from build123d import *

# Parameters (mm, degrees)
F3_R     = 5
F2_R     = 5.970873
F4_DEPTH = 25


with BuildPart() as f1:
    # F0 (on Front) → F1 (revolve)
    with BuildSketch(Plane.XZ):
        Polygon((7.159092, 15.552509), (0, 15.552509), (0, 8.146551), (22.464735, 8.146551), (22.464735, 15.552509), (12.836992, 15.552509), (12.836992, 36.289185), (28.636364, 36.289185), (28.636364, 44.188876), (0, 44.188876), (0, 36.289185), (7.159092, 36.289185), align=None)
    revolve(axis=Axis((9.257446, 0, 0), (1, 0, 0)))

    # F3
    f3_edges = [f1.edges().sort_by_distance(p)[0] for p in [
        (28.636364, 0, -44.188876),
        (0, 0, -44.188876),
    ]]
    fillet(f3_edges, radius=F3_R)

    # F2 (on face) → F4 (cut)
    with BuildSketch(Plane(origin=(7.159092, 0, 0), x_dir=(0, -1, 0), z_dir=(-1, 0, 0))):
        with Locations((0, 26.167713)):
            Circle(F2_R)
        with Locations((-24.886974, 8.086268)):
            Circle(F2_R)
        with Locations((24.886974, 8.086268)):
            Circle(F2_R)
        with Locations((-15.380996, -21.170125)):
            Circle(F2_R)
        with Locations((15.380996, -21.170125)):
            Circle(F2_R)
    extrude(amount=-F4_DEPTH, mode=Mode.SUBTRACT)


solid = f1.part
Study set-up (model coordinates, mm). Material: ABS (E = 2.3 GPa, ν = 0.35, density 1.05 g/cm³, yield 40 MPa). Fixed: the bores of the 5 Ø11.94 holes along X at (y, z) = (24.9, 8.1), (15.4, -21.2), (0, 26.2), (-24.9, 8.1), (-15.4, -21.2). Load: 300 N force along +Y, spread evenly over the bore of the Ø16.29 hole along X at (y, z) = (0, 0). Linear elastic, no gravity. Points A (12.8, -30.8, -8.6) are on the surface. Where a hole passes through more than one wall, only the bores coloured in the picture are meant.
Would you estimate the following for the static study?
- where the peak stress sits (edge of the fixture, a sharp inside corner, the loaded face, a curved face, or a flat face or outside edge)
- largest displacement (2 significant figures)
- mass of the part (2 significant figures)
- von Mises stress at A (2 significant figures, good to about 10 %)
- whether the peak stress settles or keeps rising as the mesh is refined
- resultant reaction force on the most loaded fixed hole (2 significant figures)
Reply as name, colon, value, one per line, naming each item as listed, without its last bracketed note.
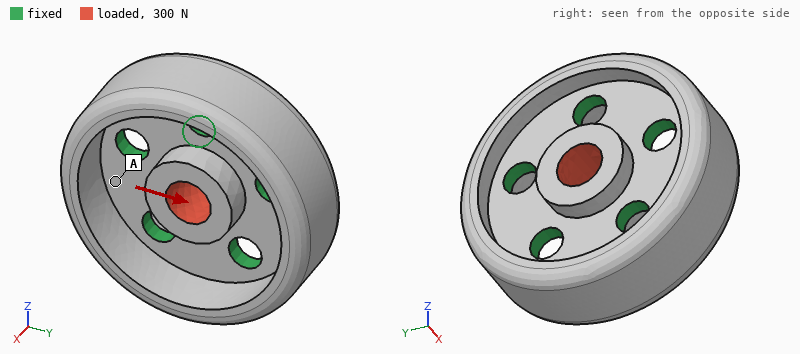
where the peak stress sits: edge of the fixture
largest displacement: 7.6 µm
mass of the part: 87 g
von Mises stress at A: 0.13 MPa
whether the peak stress settles or keeps rising as the mesh is refined: keeps rising
resultant reaction force on the most loaded fixed hole: 85 N
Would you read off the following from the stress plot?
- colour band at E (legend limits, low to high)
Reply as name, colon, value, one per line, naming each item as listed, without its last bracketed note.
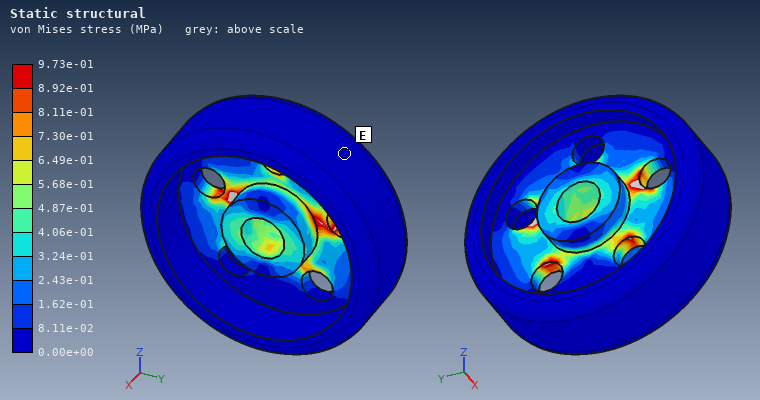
colour band at E: 0.00e+00 to 8.11e-02 MPa
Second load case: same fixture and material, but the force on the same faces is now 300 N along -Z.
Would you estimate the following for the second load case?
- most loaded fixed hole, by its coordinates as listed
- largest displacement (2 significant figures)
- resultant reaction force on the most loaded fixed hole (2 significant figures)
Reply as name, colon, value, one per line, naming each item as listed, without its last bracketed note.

most loaded fixed hole, by its coordinates as listed: (0, 26.2)
largest displacement: 7.6 µm
resultant reaction force on the most loaded fixed hole: 89 N
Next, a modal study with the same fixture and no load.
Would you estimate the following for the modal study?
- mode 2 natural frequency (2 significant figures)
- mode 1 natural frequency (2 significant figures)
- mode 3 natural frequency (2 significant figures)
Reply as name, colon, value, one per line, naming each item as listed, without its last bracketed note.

mode 2 natural frequency: 2500 Hz
mode 1 natural frequency: 2500 Hz
mode 3 natural frequency: 2900 Hz
